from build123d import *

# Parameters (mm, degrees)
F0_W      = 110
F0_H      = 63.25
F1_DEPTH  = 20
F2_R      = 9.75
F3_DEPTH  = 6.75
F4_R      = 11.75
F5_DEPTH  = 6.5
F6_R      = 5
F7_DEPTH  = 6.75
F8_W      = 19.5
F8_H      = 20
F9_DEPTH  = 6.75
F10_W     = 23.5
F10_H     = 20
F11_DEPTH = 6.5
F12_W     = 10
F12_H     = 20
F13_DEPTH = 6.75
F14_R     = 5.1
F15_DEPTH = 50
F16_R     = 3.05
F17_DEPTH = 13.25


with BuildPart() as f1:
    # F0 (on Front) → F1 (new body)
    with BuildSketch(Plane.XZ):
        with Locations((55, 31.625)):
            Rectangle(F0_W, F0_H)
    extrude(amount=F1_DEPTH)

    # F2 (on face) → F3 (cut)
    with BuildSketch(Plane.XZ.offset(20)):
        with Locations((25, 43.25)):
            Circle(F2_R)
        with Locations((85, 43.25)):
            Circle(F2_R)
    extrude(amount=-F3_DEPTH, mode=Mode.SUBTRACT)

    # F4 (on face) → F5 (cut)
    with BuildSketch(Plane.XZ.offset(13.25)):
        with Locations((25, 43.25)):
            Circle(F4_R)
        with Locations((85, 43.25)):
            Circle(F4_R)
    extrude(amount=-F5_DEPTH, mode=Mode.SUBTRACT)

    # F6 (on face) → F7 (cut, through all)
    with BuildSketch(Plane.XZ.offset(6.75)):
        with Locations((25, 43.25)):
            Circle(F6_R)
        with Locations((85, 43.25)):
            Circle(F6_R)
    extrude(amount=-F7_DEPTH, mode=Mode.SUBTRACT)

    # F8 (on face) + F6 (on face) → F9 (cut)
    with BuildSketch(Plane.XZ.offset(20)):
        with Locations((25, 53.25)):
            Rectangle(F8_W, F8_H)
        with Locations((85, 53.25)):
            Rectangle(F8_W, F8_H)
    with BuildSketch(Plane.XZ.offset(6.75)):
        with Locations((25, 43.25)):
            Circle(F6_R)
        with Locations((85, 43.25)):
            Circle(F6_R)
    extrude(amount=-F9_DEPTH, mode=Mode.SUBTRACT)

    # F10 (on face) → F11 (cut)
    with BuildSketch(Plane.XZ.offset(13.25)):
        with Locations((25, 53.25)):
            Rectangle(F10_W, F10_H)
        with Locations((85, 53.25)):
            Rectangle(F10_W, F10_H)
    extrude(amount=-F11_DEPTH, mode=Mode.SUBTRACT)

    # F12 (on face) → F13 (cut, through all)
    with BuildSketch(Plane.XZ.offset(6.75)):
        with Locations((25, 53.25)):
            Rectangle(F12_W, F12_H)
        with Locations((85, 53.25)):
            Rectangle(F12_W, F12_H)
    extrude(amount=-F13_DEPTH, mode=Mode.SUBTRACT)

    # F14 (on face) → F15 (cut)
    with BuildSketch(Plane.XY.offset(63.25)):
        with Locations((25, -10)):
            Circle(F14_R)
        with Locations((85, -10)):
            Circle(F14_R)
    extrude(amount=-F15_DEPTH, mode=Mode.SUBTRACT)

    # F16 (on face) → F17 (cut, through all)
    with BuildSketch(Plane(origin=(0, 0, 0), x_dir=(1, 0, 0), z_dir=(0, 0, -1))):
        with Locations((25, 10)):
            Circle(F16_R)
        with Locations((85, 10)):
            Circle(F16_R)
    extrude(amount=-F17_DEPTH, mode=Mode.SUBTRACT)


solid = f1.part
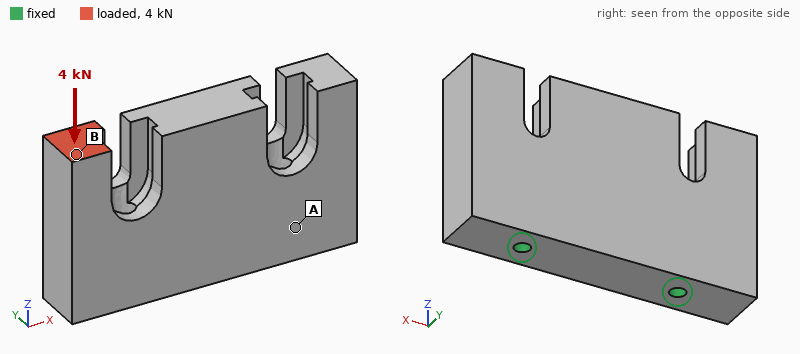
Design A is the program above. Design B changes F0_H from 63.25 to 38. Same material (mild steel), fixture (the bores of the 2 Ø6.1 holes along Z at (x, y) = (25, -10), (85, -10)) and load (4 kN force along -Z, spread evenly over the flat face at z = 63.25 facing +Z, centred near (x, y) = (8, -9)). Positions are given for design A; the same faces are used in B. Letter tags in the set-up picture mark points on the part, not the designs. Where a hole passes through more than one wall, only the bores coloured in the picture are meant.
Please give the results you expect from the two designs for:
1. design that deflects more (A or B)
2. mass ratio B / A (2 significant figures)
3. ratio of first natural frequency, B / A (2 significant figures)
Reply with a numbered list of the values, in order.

1. B
2. 0.60
3. 0.16
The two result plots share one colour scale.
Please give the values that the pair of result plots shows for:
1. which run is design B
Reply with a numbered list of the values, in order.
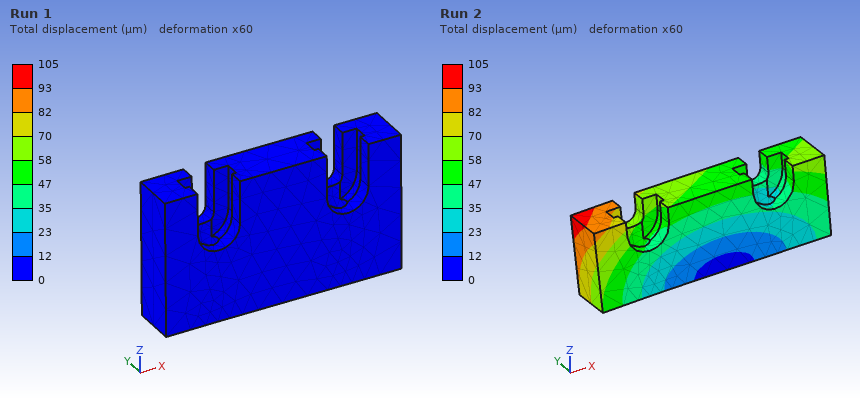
1. Run 2
